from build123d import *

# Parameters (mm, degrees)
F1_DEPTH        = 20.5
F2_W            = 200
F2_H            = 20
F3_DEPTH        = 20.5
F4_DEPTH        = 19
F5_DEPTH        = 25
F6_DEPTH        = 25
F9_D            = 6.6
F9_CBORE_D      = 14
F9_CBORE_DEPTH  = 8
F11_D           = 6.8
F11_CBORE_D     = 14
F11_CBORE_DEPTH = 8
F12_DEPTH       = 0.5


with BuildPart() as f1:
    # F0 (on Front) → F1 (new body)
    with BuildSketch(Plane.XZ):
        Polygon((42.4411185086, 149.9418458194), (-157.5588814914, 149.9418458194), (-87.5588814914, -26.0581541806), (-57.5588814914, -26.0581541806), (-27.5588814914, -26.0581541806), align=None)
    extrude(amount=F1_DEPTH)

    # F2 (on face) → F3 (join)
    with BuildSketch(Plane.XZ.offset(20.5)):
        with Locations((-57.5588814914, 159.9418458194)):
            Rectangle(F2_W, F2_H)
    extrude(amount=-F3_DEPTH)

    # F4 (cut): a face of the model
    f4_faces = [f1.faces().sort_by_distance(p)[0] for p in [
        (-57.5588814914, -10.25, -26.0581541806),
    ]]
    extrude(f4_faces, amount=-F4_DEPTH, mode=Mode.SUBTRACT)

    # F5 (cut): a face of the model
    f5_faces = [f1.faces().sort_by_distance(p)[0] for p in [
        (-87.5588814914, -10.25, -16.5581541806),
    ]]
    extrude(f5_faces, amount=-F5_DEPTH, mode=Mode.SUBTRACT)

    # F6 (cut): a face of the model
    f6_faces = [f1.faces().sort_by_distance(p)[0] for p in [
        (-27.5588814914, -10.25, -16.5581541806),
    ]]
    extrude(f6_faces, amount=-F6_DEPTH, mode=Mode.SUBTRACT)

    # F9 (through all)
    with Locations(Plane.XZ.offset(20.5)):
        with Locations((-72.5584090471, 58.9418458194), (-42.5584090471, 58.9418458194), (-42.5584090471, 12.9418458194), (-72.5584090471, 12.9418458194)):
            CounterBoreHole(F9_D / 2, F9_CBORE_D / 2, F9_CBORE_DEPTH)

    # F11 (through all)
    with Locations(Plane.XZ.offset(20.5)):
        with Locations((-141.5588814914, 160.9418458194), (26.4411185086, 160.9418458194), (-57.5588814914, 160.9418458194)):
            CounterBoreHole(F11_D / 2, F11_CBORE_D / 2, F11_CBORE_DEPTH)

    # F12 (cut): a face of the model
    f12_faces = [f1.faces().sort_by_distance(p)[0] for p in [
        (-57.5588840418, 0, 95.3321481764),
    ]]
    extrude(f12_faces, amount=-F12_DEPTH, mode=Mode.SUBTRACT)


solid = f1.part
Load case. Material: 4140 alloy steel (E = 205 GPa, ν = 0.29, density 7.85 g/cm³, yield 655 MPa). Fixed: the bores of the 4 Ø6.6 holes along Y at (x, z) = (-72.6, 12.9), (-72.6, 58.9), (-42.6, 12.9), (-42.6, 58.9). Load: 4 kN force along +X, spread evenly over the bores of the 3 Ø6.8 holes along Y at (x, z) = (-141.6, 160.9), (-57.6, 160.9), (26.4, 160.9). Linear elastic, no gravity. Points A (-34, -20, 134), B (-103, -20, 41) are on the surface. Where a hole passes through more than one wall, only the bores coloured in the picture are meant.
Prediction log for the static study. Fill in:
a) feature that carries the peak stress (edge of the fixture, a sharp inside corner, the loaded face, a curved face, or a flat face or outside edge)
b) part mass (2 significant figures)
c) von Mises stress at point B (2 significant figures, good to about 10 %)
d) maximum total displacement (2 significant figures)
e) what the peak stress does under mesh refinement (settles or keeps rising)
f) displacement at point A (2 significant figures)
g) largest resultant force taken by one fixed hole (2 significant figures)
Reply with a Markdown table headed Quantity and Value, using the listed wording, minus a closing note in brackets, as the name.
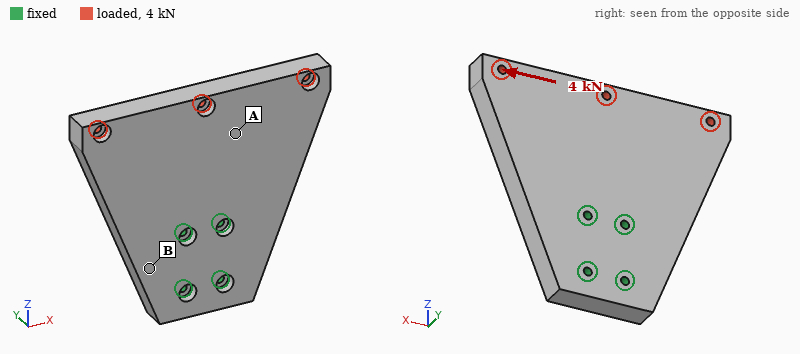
| Quantity | Value |
|---|---|
| feature that carries the peak stress | edge of the fixture |
| part mass | 3.9 kg |
| von Mises stress at point B | 6.8 MPa |
| maximum total displacement | 16 µm |
| what the peak stress does under mesh refinement | keeps rising |
| displacement at point A | 7.4 µm |
| largest resultant force taken by one fixed hole | 5.6 kN |
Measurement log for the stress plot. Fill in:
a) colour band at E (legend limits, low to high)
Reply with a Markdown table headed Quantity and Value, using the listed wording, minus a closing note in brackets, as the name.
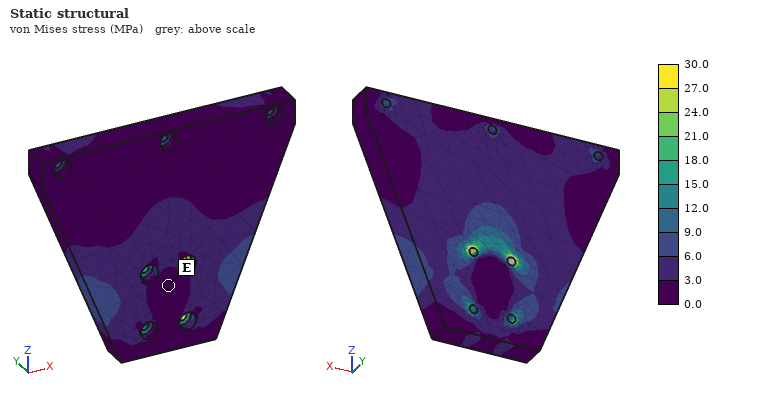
| Quantity | Value |
|---|---|
| colour band at E | 0.0 to 3.0 MPa |
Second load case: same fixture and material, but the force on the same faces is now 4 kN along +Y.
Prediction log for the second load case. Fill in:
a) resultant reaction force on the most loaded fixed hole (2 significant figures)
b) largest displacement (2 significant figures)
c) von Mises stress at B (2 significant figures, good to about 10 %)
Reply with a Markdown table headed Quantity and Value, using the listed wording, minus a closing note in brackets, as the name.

| Quantity | Value |
|---|---|
| resultant reaction force on the most loaded fixed hole | 5.9 kN |
| largest displacement | 0.14 mm |
| von Mises stress at B | 29 MPa |
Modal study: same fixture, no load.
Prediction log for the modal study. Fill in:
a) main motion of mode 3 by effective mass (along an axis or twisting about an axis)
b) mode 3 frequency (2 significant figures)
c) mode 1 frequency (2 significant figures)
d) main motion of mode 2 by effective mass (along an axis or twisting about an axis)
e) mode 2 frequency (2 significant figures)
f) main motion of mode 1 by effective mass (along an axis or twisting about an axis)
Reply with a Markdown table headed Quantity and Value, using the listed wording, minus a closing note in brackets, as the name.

| Quantity | Value |
|---|---|
| main motion of mode 3 by effective mass | along X |
| mode 3 frequency | 2400 Hz |
| mode 1 frequency | 870 Hz |
| main motion of mode 2 by effective mass | twisting about Z |
| mode 2 frequency | 1200 Hz |
| main motion of mode 1 by effective mass | along Y |
